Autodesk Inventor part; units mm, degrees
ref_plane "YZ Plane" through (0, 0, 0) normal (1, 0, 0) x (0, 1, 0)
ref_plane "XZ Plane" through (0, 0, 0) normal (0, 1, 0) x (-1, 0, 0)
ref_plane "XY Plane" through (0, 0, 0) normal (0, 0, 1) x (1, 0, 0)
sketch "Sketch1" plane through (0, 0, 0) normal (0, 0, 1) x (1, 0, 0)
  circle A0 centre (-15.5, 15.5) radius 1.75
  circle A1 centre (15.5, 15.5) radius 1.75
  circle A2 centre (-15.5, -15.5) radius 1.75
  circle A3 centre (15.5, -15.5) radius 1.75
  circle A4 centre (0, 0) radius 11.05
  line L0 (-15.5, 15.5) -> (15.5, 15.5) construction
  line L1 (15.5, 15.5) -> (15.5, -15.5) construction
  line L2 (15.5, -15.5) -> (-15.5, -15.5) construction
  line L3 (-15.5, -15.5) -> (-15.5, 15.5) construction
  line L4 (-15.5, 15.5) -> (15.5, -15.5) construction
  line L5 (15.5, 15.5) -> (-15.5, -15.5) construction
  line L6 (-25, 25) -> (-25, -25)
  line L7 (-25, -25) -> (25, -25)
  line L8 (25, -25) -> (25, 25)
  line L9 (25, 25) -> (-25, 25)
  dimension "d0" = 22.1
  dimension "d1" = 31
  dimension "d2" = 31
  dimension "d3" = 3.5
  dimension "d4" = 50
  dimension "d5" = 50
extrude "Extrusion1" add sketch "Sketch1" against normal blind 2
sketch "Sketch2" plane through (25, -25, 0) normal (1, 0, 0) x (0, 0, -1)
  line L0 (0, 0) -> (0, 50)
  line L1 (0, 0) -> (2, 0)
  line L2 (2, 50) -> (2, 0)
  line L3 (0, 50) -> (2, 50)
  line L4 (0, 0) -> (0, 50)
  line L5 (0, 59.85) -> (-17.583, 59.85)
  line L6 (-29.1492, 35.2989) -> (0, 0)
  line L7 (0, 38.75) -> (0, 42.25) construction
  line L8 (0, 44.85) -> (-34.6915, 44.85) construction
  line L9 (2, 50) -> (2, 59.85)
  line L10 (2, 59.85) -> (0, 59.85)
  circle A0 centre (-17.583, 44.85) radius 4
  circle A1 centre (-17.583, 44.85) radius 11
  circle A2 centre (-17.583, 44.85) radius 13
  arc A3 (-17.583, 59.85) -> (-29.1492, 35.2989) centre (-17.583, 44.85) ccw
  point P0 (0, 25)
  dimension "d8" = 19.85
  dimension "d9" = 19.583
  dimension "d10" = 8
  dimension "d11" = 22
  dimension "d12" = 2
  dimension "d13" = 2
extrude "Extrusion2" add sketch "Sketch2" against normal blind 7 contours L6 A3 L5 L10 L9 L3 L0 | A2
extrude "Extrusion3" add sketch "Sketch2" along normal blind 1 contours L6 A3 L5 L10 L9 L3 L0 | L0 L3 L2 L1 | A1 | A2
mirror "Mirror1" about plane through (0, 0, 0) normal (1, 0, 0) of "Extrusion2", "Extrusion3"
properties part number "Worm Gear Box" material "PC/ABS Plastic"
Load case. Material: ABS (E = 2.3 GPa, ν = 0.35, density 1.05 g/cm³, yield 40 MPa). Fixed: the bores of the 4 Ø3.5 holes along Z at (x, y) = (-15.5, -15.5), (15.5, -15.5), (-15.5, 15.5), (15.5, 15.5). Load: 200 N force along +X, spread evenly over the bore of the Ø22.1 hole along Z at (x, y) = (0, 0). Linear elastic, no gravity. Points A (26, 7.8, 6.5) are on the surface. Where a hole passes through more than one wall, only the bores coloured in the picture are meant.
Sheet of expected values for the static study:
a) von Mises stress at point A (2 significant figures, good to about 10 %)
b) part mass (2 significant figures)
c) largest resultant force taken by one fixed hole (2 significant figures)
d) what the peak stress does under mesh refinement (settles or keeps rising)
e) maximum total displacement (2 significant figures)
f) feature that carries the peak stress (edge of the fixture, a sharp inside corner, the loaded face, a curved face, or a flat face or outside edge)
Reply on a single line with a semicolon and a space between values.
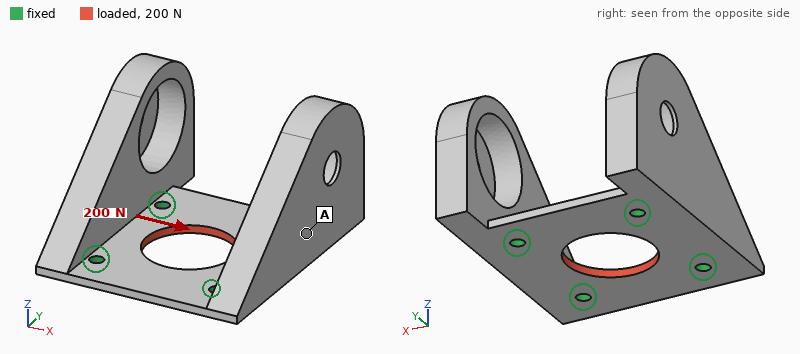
0.37 MPa; 20 g; 50 N; keeps rising; 18 µm; edge of the fixture
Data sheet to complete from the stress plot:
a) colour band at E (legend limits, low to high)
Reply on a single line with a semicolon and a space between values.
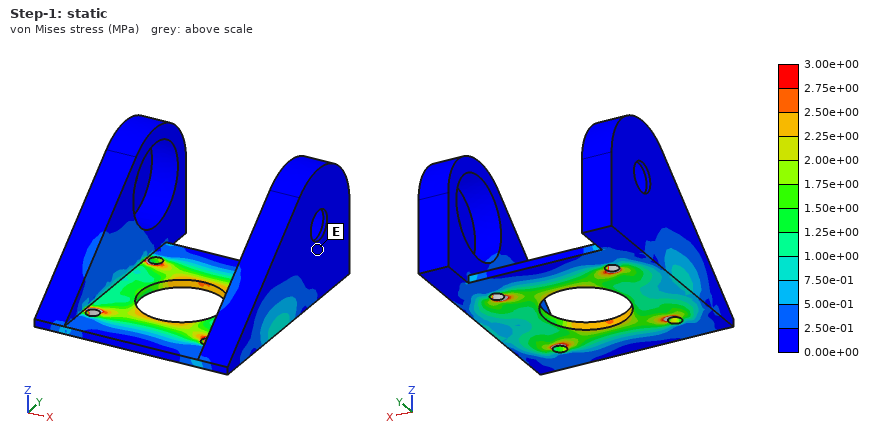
0.00e+00 to 2.50e-01 MPa
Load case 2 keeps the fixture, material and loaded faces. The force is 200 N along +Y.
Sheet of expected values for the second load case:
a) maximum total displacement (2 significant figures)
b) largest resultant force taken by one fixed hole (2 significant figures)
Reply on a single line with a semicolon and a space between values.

20 µm; 52 N
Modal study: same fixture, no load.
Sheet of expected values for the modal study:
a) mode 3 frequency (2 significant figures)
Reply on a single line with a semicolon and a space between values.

1900 Hz
